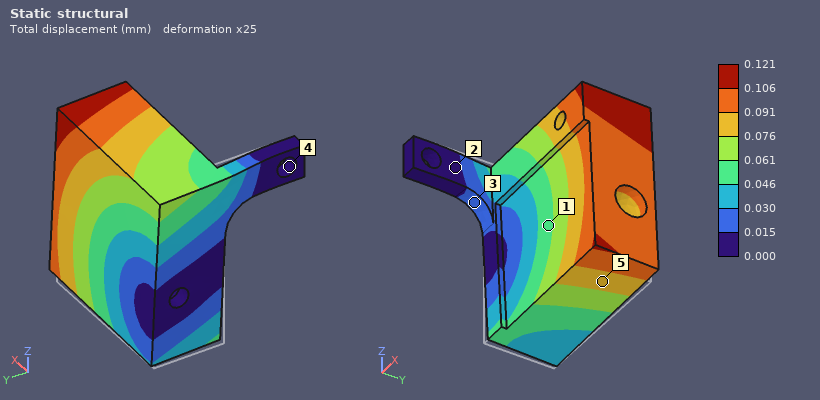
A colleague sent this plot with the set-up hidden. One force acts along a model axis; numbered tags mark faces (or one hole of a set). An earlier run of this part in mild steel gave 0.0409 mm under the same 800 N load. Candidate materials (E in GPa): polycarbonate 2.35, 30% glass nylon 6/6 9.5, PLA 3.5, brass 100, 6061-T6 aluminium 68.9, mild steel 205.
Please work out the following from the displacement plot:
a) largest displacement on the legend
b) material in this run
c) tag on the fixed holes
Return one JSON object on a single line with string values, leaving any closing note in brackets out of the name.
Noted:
{"largest displacement on the legend": "0.121 mm", "material in this run": "6061-T6 aluminium", "tag on the fixed holes": "4"}
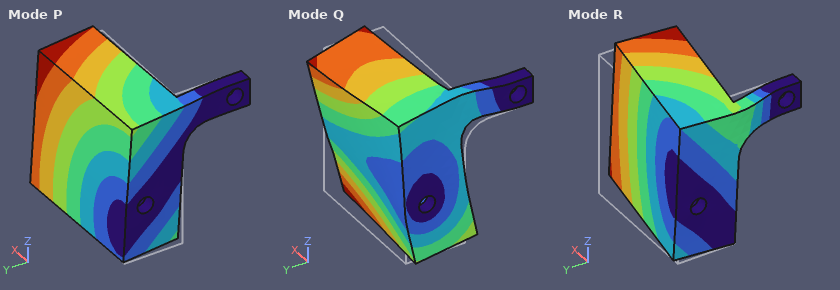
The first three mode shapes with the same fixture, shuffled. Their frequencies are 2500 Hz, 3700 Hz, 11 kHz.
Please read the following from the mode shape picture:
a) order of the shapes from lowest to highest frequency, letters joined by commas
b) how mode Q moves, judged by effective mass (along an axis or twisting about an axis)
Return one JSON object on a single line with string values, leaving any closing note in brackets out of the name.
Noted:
{"order of the shapes from lowest to highest frequency, letters joined by commas": "P, R, Q", "how mode Q moves, judged by effective mass": "twisting about X"}
